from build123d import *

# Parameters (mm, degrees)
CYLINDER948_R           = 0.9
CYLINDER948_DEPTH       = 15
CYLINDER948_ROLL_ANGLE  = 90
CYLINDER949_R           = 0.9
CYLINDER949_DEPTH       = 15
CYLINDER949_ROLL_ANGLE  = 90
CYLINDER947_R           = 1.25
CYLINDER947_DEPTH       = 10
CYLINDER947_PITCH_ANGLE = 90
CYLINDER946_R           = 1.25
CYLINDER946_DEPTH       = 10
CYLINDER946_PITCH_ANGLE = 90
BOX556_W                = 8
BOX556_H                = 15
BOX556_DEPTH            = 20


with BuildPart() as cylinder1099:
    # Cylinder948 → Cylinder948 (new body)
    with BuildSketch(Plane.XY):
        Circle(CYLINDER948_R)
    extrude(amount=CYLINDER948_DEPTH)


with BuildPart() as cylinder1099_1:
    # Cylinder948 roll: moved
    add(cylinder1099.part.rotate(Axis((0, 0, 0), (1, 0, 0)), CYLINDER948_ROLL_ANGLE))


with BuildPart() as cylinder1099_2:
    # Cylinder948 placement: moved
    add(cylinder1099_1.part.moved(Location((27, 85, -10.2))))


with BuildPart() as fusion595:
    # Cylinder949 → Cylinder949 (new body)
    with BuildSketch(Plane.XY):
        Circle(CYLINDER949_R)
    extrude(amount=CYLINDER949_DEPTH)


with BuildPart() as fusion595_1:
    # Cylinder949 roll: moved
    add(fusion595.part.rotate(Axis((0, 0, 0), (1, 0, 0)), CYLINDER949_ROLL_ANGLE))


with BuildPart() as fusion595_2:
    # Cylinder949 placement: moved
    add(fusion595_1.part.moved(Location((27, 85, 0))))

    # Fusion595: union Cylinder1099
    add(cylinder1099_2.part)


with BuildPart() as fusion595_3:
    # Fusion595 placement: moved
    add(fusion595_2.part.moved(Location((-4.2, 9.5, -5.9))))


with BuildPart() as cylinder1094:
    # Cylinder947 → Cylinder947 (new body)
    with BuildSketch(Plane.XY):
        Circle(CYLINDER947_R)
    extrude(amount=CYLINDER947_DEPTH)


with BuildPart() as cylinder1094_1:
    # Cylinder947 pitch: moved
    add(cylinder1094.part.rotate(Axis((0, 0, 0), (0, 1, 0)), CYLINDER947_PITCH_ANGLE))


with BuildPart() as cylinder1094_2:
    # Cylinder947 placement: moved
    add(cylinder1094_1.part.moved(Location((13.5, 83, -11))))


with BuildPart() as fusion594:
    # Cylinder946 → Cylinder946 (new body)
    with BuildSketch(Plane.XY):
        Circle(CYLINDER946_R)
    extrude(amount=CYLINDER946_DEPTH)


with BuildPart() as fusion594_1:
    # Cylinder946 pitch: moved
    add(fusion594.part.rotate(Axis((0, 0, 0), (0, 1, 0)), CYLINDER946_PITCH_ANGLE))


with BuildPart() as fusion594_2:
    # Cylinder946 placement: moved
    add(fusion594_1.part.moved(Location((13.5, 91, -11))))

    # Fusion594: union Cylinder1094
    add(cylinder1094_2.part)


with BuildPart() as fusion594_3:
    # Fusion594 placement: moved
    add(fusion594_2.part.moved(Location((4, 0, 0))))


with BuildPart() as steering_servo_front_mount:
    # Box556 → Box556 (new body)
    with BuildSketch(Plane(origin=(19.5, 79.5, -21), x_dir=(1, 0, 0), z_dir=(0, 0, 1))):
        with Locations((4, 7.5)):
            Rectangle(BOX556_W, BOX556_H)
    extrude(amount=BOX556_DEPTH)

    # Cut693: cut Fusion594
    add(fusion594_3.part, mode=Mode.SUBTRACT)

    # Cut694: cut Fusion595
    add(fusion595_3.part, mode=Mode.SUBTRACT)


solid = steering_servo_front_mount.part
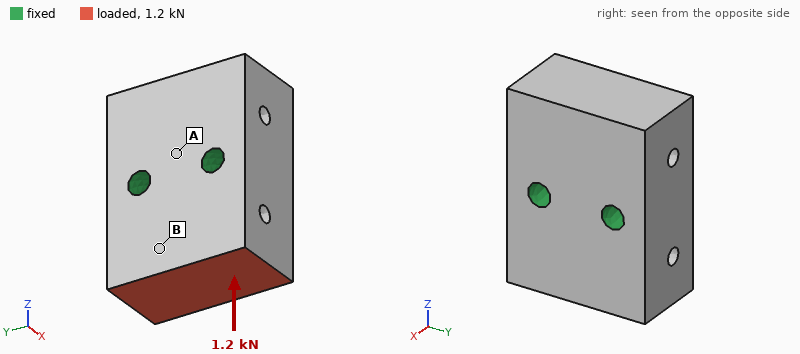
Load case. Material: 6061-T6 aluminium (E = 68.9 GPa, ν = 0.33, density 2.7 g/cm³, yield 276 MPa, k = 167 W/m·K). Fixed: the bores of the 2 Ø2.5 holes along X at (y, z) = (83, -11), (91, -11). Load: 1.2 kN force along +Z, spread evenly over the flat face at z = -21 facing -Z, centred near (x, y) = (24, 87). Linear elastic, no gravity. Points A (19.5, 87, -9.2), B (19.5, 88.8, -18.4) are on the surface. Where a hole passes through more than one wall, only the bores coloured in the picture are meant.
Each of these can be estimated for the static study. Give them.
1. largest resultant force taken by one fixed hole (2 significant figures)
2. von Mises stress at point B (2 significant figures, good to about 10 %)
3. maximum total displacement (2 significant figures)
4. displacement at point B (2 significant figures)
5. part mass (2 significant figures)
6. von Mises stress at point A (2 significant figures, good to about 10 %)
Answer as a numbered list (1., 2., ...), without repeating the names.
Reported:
1. 610 N
2. 11 MPa
3. 1.8 µm
4. 1.2 µm
5. 6.1 g
6. 3.5 MPa
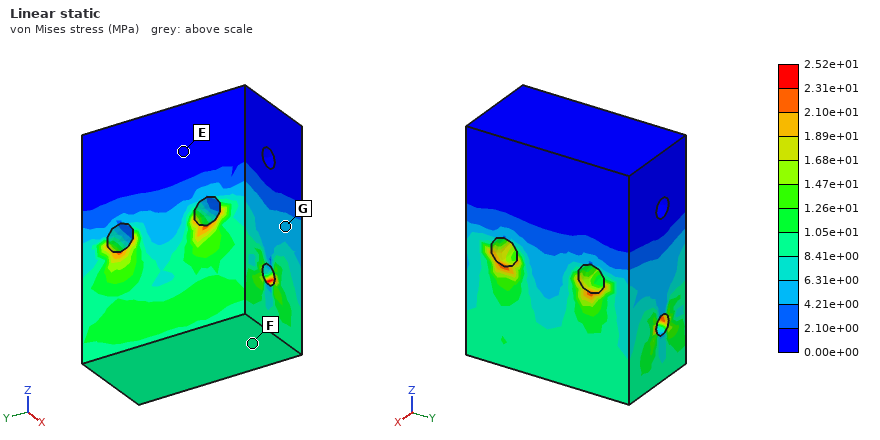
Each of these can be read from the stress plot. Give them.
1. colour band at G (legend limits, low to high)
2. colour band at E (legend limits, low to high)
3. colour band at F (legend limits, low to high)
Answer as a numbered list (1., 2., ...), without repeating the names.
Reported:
1. 4.21e+00 to 6.31e+00 MPa
2. 0.00e+00 to 2.10e+00 MPa
3. 8.41e+00 to 1.05e+01 MPa
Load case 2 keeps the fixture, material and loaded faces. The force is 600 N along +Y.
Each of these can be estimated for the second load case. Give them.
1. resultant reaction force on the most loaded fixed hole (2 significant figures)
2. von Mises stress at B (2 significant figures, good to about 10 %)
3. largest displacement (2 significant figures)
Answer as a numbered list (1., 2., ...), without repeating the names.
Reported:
1. 670 N
2. 15 MPa
3. 5.0 µm
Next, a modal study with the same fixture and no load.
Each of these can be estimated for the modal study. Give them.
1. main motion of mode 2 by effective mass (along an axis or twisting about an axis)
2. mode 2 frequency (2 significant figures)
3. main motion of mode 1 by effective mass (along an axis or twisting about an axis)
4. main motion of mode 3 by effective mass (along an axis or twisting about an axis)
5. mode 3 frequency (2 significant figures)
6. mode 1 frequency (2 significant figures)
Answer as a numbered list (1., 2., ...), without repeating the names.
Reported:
1. along X
2. 50 kHz
3. twisting about Y
4. twisting about X
5. 54 kHz
6. 45 kHz
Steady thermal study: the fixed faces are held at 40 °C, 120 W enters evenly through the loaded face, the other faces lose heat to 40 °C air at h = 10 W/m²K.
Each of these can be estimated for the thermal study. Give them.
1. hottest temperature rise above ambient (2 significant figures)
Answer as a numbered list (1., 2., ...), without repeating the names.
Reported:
1. 62 K
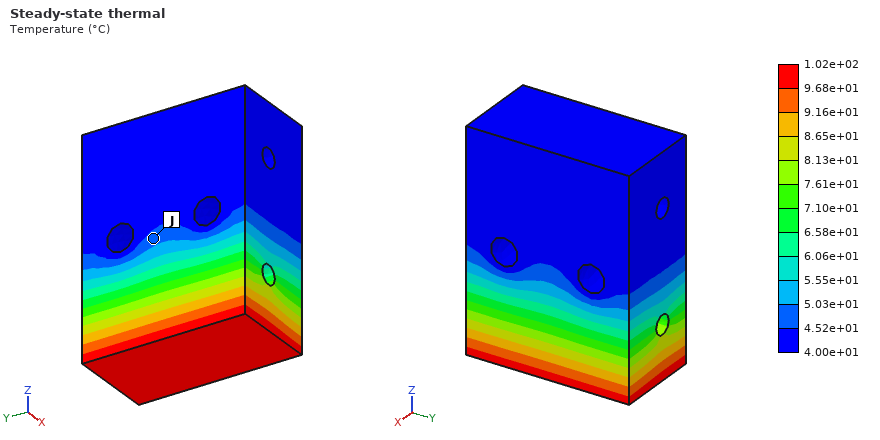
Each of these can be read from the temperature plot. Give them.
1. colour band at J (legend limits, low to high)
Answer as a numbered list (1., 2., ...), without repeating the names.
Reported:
1. 4.52e+01 to 5.03e+01 °C
